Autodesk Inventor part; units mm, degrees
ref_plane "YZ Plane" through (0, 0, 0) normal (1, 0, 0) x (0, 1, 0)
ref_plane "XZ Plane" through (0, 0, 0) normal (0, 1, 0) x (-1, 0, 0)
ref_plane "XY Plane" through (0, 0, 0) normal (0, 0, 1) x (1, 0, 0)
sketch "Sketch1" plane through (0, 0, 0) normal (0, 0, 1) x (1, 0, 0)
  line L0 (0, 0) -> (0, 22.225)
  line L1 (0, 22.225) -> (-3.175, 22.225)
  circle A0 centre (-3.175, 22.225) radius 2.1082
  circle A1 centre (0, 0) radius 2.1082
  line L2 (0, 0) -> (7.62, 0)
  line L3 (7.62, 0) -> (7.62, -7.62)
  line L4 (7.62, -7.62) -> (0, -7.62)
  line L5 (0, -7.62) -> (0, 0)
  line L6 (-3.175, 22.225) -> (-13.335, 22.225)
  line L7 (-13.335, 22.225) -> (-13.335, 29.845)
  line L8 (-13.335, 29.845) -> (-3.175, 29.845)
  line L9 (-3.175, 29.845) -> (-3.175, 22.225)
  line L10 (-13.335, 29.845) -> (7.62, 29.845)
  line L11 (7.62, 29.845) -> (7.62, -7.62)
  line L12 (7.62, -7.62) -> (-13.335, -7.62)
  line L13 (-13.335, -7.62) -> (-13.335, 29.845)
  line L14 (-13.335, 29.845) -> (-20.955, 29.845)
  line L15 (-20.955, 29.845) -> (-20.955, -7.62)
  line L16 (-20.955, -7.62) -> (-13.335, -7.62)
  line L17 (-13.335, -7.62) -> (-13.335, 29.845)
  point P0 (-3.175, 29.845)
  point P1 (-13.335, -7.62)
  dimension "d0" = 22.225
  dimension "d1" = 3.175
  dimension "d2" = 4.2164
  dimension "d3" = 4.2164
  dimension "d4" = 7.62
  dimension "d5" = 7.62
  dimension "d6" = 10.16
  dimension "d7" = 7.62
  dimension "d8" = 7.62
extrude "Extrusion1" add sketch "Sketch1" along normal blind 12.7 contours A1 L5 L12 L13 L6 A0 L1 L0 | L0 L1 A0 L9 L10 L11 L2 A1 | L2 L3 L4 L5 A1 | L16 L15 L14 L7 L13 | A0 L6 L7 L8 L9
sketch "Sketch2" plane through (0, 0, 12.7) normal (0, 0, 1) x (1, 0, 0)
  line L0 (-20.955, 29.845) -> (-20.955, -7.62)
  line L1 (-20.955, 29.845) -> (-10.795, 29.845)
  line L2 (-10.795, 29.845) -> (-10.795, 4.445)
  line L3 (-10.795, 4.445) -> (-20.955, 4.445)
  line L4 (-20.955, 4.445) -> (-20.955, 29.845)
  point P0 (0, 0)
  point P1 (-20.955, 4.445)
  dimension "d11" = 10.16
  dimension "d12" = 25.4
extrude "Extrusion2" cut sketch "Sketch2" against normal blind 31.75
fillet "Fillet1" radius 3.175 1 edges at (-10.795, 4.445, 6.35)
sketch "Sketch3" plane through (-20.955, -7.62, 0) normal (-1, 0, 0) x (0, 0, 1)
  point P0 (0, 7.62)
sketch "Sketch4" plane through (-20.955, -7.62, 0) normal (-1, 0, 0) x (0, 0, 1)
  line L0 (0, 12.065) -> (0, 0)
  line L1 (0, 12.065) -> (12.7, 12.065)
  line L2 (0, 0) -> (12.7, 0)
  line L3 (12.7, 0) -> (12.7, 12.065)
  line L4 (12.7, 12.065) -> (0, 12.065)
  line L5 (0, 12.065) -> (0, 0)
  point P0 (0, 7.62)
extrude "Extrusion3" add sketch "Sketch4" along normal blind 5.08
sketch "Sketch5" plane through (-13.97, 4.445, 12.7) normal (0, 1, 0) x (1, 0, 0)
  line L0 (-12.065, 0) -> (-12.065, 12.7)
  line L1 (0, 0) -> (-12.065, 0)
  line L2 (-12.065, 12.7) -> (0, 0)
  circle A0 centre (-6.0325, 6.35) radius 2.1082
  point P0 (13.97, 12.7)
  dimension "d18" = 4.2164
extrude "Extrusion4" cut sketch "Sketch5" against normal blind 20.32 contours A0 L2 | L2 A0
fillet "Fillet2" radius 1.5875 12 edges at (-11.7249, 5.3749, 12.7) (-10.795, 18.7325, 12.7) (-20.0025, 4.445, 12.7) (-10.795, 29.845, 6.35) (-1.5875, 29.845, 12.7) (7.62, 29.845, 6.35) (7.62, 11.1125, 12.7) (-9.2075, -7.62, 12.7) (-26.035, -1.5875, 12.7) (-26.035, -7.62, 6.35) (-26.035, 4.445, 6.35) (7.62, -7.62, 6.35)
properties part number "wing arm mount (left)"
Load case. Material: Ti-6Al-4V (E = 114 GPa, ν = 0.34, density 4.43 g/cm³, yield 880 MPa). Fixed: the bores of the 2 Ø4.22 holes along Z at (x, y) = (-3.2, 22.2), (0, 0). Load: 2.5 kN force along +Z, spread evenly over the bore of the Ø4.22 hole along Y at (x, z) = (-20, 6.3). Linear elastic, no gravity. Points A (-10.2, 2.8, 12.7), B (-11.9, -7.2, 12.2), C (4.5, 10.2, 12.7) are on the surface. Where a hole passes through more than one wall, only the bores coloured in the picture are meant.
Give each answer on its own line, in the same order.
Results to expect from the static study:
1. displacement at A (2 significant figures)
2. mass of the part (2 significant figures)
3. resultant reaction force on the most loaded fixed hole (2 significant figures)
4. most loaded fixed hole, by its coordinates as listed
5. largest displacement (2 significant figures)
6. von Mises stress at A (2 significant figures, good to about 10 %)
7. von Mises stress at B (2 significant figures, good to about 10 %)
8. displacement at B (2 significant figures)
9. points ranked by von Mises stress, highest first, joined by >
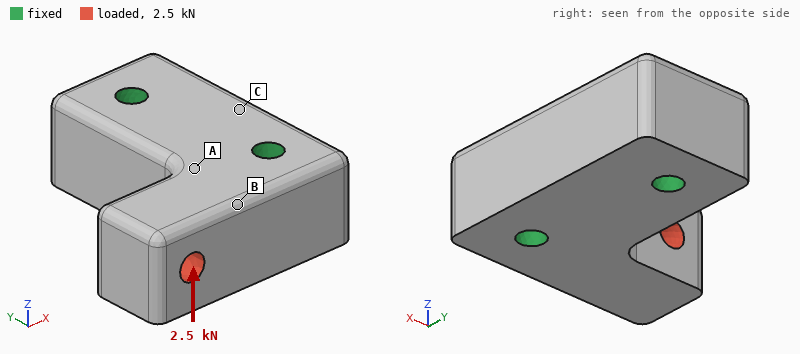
13 µm
46 g
2.3 kN
(0, 0)
45 µm
82 MPa
51 MPa
16 µm
A > B > C
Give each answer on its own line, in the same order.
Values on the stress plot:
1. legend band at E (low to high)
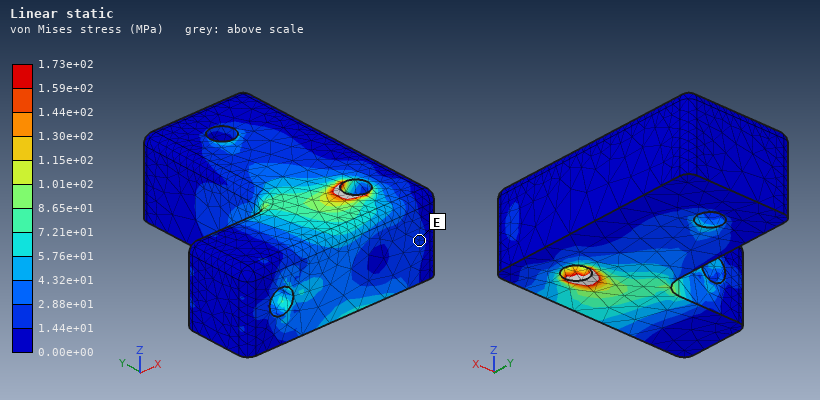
1.44e+01 to 2.88e+01 MPa
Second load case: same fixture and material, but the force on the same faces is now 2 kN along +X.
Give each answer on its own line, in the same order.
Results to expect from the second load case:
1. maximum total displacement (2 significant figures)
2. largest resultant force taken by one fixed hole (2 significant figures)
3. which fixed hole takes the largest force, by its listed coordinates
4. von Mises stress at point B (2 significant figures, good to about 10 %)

4.5 µm
2.0 kN
(0, 0)
14 MPa
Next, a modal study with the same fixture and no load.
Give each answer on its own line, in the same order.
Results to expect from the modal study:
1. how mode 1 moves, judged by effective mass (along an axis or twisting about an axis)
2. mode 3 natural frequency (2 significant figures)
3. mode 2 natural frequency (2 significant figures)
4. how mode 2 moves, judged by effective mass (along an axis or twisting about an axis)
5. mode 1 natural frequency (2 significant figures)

along Z
35 kHz
18 kHz
along Y
15 kHz
